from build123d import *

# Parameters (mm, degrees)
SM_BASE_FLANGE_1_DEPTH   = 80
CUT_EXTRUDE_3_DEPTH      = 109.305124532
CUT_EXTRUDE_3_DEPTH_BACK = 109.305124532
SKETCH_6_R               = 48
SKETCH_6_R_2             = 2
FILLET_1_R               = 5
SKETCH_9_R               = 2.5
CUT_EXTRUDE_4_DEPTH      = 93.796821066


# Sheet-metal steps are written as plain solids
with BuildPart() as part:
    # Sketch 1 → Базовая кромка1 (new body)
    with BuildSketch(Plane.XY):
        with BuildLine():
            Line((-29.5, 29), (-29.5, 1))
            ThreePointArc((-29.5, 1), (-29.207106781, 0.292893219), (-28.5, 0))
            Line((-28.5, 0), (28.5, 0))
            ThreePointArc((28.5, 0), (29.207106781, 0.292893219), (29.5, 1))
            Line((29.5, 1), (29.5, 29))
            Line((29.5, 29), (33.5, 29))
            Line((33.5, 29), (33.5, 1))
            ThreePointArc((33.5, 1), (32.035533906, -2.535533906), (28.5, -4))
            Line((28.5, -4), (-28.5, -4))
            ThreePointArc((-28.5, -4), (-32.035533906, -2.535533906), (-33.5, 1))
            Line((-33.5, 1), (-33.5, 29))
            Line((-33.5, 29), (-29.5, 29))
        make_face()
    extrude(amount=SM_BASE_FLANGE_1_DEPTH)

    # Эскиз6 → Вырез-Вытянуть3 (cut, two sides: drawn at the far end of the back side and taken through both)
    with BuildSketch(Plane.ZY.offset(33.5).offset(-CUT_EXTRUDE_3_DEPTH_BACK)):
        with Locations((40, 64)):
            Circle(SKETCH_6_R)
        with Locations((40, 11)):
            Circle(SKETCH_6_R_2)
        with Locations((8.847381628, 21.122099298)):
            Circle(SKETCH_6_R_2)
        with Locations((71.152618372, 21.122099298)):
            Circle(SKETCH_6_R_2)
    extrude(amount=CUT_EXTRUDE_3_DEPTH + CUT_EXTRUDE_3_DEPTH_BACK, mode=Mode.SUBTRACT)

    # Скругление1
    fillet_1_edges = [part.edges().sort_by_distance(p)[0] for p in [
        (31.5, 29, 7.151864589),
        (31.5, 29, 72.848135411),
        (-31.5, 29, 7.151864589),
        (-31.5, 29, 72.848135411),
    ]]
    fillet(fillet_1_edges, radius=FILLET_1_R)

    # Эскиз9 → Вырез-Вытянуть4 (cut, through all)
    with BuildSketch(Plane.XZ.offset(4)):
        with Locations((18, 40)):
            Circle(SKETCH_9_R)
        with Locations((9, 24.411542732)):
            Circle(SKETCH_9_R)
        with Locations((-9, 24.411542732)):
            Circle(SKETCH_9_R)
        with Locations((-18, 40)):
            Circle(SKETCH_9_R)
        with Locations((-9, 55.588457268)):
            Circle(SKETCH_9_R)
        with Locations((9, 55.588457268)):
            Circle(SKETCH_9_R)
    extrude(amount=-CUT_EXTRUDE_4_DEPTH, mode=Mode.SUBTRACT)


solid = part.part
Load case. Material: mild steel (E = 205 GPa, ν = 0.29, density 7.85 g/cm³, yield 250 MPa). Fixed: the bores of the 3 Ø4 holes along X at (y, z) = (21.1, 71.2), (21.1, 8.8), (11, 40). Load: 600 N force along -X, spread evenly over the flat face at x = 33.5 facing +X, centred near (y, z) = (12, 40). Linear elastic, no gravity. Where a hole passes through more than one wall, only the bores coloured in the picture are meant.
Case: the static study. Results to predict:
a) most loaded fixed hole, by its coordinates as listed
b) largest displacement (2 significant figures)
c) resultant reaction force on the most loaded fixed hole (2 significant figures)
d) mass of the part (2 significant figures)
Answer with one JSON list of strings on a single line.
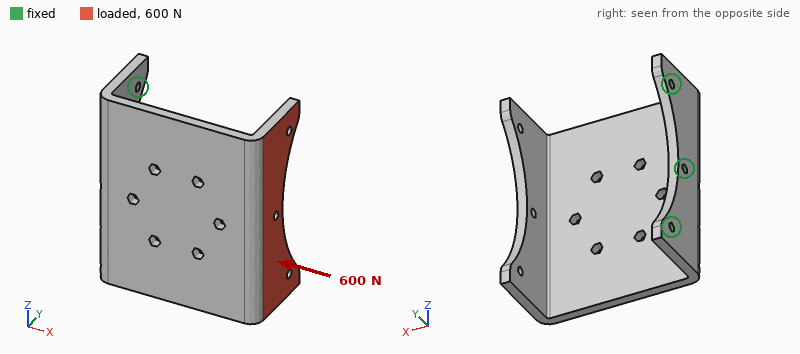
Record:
["(11, 40)", "0.31 mm", "340 N", "260 g"]
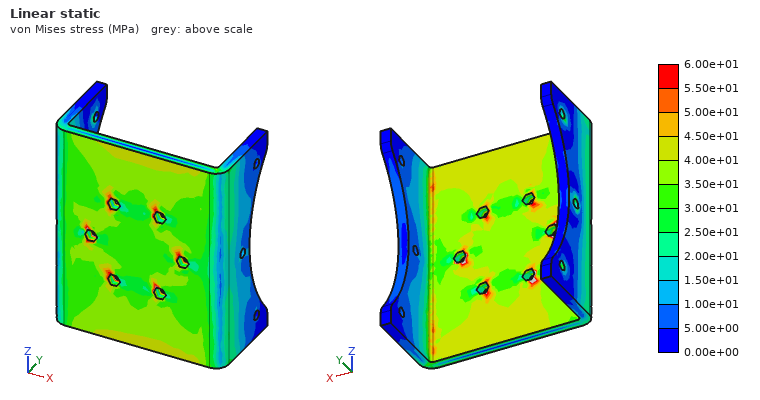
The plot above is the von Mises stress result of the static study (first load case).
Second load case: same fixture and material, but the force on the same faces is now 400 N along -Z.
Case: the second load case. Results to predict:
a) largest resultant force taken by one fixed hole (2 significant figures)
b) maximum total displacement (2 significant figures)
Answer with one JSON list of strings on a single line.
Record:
["360 N", "0.21 mm"]
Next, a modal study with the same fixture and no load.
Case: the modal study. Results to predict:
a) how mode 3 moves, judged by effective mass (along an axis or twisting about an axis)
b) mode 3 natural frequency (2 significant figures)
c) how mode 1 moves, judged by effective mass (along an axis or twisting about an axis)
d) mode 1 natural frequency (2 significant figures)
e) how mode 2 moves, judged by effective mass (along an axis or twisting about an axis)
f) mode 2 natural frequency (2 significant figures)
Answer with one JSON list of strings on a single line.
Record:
["along Z", "1400 Hz", "along Y", "390 Hz", "along Z", "790 Hz"]
